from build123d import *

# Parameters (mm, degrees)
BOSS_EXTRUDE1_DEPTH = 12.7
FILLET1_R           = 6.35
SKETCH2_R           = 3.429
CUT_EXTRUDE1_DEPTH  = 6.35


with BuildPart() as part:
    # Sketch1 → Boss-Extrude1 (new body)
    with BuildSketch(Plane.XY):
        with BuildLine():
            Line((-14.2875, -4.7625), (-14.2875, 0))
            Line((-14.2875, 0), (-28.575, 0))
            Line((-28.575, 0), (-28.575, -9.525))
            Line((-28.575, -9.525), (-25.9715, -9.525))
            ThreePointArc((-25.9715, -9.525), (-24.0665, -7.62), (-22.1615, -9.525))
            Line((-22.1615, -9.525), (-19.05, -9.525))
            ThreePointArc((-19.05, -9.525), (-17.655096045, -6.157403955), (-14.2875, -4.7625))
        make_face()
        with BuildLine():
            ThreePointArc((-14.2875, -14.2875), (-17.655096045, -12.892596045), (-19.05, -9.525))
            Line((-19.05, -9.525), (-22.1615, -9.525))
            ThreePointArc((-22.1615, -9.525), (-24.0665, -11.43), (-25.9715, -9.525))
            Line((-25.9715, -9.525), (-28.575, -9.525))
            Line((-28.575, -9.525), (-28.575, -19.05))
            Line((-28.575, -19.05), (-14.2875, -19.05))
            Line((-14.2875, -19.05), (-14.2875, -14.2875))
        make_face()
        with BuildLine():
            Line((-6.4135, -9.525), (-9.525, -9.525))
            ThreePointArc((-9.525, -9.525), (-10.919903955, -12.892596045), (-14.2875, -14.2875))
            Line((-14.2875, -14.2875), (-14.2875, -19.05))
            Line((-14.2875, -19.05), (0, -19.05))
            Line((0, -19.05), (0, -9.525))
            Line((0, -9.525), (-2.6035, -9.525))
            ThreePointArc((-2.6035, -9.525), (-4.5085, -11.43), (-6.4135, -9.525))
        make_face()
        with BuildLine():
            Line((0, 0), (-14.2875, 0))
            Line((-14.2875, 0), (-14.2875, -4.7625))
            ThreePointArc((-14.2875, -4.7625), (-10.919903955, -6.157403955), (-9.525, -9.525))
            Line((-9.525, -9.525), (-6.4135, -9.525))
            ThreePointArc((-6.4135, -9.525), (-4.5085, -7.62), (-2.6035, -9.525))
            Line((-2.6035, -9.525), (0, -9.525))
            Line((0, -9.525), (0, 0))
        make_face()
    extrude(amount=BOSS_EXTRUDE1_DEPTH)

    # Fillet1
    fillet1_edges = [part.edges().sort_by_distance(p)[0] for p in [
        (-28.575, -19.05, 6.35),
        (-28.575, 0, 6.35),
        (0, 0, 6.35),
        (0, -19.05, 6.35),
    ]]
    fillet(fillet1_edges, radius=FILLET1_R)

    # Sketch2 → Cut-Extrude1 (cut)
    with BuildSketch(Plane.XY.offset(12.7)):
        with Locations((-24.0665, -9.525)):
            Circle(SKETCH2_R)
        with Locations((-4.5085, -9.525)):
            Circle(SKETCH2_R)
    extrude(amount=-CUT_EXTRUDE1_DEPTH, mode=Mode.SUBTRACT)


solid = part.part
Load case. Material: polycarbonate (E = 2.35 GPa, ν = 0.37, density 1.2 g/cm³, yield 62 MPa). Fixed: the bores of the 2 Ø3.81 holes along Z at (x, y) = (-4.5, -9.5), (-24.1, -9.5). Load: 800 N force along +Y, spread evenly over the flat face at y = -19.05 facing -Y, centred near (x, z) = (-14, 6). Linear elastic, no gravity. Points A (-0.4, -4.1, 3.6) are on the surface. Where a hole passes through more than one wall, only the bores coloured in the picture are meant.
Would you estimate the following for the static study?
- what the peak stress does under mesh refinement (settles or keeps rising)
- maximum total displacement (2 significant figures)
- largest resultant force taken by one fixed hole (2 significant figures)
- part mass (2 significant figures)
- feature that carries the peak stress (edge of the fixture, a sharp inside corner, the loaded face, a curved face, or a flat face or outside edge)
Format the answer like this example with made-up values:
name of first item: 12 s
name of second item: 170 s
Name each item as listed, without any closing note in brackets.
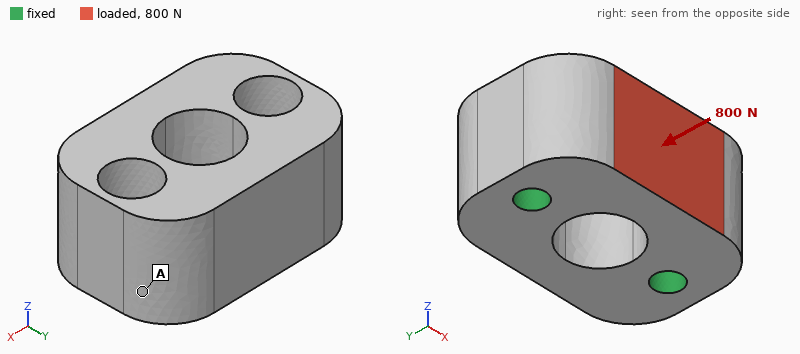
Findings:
what the peak stress does under mesh refinement: keeps rising
maximum total displacement: 0.13 mm
largest resultant force taken by one fixed hole: 420 N
part mass: 5.9 g
feature that carries the peak stress: edge of the fixture
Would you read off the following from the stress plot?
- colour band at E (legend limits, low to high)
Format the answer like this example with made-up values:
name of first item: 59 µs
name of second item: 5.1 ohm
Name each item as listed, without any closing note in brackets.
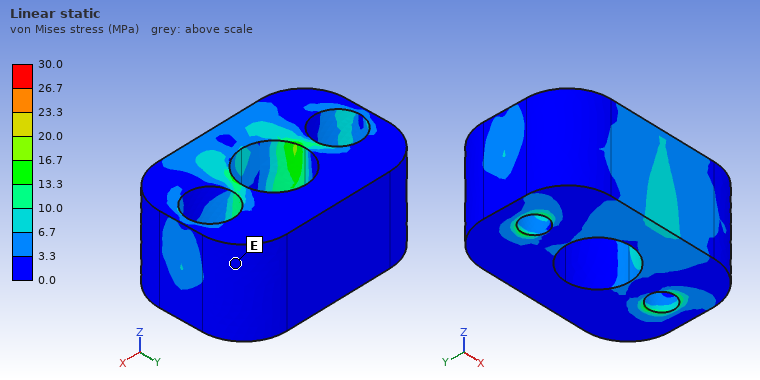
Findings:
colour band at E: 0.0 to 3.3 MPa
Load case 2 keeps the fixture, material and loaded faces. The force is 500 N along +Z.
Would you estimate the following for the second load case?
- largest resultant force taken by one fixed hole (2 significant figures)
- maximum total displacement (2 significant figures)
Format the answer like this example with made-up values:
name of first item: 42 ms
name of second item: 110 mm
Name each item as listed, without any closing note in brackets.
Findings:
largest resultant force taken by one fixed hole: 260 N
maximum total displacement: 0.19 mm
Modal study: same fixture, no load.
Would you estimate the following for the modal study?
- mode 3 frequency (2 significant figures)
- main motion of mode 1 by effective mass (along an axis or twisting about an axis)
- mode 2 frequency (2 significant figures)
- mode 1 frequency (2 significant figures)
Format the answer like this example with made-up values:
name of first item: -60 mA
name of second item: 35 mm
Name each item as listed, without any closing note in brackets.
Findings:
mode 3 frequency: 12 kHz
main motion of mode 1 by effective mass: along Y
mode 2 frequency: 11 kHz
mode 1 frequency: 6600 Hz
